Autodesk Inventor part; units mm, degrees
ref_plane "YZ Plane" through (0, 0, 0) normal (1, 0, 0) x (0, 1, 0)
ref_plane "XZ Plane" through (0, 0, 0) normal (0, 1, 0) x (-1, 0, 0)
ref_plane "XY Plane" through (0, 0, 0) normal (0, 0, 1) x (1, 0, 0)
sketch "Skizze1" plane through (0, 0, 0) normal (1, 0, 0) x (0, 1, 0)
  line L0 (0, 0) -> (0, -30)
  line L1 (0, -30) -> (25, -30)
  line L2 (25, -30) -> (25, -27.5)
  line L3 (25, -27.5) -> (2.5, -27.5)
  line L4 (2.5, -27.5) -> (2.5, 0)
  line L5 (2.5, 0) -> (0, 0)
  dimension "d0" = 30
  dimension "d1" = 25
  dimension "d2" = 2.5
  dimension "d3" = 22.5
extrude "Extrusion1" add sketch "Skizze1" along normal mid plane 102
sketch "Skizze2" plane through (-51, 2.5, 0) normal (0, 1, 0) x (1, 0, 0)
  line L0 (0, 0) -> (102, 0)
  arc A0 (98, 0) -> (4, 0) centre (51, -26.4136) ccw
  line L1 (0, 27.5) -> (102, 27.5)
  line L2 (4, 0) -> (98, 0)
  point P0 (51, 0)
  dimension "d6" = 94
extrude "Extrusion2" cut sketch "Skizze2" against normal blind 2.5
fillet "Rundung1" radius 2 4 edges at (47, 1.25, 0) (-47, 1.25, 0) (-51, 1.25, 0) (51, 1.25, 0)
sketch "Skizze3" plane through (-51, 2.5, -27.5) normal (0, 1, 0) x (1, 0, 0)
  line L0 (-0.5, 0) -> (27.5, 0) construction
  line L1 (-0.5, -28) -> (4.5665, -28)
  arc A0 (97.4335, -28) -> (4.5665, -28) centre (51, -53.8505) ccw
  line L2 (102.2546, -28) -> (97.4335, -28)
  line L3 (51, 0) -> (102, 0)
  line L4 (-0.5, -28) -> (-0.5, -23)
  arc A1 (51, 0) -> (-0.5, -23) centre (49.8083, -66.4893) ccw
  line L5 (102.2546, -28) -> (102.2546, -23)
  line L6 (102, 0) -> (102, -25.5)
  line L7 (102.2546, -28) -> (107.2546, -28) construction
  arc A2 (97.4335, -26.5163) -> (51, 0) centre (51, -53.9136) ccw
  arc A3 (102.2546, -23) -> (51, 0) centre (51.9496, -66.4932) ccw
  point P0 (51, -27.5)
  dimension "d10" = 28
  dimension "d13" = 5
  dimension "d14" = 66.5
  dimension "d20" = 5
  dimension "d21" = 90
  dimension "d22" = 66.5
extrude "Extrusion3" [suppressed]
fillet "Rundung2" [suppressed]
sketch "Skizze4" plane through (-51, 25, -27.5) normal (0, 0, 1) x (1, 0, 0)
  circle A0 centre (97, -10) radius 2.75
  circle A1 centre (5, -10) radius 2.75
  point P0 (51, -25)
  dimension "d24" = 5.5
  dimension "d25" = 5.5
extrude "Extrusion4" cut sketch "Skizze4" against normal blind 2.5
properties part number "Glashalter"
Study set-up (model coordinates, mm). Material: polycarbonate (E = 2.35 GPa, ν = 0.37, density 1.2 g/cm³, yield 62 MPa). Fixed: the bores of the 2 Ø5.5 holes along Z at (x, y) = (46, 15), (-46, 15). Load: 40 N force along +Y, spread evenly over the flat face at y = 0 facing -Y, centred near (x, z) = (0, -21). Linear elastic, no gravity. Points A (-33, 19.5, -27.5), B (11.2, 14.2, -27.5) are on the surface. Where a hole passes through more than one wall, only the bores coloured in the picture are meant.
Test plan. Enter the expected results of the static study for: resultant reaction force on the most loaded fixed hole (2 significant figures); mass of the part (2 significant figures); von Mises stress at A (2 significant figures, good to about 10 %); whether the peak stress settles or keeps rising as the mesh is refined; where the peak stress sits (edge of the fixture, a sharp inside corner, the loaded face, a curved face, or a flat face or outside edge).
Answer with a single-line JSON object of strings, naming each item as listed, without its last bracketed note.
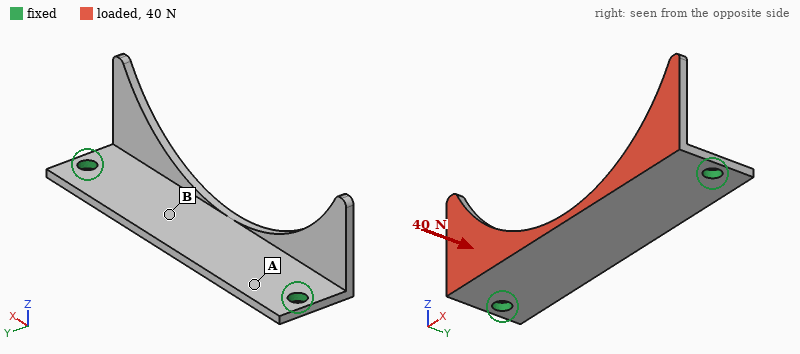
{"resultant reaction force on the most loaded fixed hole": "20 N", "mass of the part": "10 g", "von Mises stress at A": "2.5 MPa", "whether the peak stress settles or keeps rising as the mesh is refined": "keeps rising", "where the peak stress sits": "edge of the fixture"}
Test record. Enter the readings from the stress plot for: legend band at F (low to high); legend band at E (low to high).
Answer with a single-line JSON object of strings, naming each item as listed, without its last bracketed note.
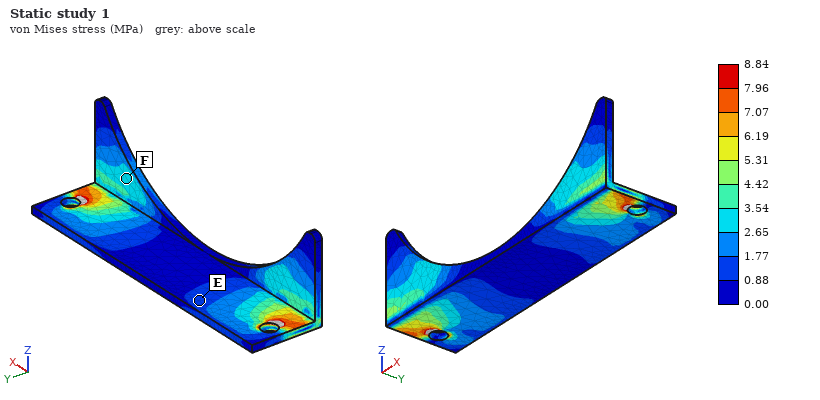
{"legend band at F": "2.65 to 3.54 MPa", "legend band at E": "0.88 to 1.77 MPa"}
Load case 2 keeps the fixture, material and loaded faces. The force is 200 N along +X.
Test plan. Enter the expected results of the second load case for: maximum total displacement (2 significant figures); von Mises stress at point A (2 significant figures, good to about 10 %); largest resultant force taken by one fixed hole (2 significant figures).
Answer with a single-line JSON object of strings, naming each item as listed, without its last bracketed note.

{"maximum total displacement": "0.62 mm", "von Mises stress at point A": "1.7 MPa", "largest resultant force taken by one fixed hole": "110 N"}
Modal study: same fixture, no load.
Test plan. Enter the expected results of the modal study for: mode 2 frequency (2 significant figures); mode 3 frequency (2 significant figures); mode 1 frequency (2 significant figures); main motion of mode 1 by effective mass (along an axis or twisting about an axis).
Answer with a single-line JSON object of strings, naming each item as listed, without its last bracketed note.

{"mode 2 frequency": "600 Hz", "mode 3 frequency": "680 Hz", "mode 1 frequency": "440 Hz", "main motion of mode 1 by effective mass": "along Z"}
